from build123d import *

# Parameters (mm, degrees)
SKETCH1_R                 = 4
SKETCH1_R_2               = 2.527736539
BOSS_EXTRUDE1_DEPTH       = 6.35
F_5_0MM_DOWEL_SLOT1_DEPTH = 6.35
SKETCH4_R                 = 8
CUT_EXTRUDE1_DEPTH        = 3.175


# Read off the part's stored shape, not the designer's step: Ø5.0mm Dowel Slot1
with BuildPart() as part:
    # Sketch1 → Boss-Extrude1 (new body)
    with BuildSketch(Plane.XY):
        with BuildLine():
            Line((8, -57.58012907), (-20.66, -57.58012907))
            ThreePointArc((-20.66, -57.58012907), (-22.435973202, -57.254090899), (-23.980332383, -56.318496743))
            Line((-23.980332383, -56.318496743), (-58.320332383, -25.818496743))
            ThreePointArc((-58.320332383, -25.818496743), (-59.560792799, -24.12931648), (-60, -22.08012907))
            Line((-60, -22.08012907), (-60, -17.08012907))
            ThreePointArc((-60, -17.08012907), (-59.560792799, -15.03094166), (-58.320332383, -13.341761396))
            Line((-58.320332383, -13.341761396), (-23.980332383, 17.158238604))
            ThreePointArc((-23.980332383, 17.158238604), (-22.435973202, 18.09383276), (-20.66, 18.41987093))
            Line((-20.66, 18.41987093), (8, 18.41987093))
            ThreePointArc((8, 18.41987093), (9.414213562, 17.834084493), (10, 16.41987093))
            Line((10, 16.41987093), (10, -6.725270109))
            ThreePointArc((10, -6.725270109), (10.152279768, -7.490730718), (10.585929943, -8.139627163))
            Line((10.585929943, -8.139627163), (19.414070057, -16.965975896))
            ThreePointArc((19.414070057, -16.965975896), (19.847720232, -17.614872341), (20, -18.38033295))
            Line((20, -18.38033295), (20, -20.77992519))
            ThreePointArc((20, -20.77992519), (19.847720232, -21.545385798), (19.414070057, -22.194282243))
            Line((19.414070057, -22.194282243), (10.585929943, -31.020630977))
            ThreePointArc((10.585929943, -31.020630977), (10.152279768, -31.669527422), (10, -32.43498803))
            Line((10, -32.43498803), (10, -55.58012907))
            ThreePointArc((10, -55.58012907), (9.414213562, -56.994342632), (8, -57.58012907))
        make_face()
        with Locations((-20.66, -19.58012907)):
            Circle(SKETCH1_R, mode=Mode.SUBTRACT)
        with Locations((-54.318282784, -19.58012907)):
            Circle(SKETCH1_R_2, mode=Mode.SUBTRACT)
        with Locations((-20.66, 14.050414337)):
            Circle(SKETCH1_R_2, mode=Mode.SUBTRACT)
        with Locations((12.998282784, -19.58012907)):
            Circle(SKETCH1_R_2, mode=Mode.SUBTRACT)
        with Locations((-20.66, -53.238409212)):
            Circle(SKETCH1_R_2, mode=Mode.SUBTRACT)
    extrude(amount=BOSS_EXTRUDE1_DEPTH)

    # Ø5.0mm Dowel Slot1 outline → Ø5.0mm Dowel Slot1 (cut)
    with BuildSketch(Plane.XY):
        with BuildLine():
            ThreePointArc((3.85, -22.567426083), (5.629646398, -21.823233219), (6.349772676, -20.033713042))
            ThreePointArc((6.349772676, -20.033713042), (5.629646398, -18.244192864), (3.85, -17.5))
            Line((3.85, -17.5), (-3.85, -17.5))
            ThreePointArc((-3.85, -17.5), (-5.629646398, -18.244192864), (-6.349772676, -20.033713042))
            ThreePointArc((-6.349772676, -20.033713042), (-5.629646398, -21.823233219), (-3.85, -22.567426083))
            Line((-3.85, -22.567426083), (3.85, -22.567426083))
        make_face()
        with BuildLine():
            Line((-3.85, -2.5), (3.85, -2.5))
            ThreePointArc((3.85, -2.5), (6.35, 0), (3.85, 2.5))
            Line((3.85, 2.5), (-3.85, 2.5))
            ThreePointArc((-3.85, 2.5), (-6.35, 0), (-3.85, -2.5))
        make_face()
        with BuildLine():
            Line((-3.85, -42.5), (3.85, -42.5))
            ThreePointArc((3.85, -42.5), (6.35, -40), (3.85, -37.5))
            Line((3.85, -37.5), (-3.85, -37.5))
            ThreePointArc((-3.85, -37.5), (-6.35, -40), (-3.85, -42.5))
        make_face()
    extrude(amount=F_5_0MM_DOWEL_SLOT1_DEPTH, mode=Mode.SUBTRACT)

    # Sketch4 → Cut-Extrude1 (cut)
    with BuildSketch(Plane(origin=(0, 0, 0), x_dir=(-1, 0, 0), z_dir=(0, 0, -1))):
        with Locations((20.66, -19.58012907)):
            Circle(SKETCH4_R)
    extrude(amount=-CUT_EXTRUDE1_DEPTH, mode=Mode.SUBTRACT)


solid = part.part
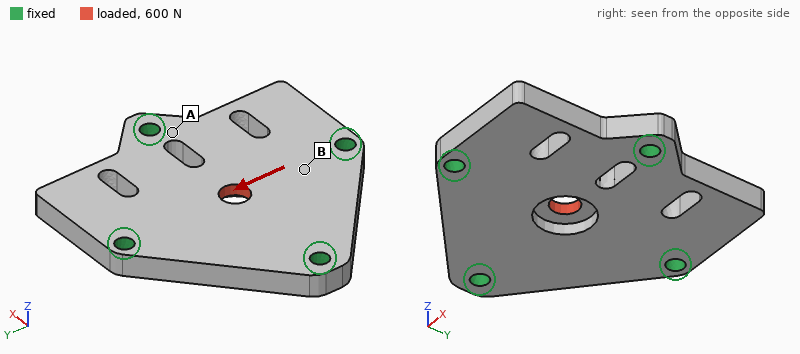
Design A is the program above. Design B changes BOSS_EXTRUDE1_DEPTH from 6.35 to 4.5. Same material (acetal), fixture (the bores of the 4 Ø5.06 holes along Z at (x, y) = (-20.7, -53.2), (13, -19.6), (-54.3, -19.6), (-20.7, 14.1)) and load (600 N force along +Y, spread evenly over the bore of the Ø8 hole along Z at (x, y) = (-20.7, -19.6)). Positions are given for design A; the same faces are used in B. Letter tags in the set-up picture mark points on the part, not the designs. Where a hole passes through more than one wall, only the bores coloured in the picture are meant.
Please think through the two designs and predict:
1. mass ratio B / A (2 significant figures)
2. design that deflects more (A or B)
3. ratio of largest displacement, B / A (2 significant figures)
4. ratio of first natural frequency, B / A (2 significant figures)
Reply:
0.70
B
1.9
0.76
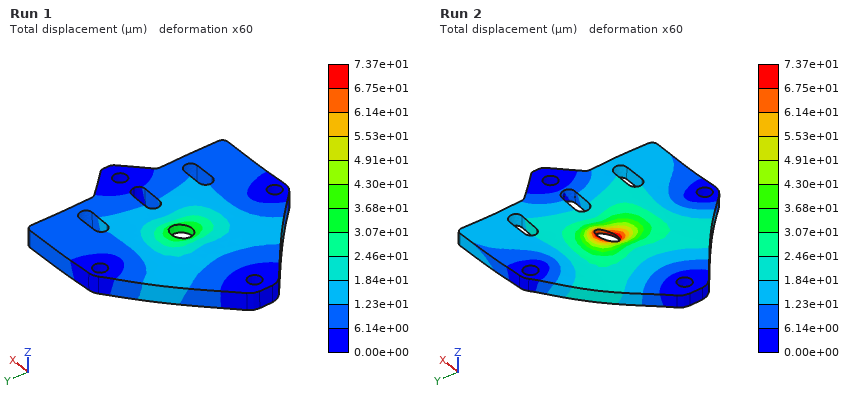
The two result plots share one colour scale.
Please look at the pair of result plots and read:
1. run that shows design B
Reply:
Run 2
